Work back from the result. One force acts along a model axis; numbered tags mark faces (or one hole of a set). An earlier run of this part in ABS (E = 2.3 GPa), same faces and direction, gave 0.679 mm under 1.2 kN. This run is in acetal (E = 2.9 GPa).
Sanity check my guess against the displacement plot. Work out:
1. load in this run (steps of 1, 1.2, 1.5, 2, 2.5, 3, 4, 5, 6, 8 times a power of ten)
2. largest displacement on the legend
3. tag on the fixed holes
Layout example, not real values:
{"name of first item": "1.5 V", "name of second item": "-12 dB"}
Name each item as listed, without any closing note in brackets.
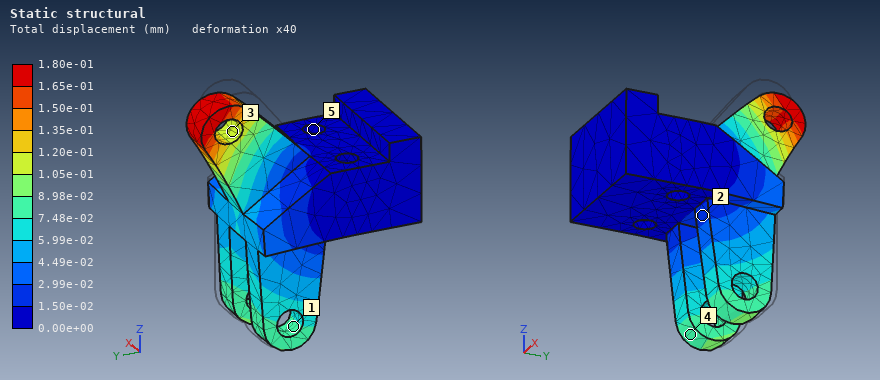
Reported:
{"load in this run": "400 N", "largest displacement on the legend": "1.80e-01 mm", "tag on the fixed holes": "5"}
